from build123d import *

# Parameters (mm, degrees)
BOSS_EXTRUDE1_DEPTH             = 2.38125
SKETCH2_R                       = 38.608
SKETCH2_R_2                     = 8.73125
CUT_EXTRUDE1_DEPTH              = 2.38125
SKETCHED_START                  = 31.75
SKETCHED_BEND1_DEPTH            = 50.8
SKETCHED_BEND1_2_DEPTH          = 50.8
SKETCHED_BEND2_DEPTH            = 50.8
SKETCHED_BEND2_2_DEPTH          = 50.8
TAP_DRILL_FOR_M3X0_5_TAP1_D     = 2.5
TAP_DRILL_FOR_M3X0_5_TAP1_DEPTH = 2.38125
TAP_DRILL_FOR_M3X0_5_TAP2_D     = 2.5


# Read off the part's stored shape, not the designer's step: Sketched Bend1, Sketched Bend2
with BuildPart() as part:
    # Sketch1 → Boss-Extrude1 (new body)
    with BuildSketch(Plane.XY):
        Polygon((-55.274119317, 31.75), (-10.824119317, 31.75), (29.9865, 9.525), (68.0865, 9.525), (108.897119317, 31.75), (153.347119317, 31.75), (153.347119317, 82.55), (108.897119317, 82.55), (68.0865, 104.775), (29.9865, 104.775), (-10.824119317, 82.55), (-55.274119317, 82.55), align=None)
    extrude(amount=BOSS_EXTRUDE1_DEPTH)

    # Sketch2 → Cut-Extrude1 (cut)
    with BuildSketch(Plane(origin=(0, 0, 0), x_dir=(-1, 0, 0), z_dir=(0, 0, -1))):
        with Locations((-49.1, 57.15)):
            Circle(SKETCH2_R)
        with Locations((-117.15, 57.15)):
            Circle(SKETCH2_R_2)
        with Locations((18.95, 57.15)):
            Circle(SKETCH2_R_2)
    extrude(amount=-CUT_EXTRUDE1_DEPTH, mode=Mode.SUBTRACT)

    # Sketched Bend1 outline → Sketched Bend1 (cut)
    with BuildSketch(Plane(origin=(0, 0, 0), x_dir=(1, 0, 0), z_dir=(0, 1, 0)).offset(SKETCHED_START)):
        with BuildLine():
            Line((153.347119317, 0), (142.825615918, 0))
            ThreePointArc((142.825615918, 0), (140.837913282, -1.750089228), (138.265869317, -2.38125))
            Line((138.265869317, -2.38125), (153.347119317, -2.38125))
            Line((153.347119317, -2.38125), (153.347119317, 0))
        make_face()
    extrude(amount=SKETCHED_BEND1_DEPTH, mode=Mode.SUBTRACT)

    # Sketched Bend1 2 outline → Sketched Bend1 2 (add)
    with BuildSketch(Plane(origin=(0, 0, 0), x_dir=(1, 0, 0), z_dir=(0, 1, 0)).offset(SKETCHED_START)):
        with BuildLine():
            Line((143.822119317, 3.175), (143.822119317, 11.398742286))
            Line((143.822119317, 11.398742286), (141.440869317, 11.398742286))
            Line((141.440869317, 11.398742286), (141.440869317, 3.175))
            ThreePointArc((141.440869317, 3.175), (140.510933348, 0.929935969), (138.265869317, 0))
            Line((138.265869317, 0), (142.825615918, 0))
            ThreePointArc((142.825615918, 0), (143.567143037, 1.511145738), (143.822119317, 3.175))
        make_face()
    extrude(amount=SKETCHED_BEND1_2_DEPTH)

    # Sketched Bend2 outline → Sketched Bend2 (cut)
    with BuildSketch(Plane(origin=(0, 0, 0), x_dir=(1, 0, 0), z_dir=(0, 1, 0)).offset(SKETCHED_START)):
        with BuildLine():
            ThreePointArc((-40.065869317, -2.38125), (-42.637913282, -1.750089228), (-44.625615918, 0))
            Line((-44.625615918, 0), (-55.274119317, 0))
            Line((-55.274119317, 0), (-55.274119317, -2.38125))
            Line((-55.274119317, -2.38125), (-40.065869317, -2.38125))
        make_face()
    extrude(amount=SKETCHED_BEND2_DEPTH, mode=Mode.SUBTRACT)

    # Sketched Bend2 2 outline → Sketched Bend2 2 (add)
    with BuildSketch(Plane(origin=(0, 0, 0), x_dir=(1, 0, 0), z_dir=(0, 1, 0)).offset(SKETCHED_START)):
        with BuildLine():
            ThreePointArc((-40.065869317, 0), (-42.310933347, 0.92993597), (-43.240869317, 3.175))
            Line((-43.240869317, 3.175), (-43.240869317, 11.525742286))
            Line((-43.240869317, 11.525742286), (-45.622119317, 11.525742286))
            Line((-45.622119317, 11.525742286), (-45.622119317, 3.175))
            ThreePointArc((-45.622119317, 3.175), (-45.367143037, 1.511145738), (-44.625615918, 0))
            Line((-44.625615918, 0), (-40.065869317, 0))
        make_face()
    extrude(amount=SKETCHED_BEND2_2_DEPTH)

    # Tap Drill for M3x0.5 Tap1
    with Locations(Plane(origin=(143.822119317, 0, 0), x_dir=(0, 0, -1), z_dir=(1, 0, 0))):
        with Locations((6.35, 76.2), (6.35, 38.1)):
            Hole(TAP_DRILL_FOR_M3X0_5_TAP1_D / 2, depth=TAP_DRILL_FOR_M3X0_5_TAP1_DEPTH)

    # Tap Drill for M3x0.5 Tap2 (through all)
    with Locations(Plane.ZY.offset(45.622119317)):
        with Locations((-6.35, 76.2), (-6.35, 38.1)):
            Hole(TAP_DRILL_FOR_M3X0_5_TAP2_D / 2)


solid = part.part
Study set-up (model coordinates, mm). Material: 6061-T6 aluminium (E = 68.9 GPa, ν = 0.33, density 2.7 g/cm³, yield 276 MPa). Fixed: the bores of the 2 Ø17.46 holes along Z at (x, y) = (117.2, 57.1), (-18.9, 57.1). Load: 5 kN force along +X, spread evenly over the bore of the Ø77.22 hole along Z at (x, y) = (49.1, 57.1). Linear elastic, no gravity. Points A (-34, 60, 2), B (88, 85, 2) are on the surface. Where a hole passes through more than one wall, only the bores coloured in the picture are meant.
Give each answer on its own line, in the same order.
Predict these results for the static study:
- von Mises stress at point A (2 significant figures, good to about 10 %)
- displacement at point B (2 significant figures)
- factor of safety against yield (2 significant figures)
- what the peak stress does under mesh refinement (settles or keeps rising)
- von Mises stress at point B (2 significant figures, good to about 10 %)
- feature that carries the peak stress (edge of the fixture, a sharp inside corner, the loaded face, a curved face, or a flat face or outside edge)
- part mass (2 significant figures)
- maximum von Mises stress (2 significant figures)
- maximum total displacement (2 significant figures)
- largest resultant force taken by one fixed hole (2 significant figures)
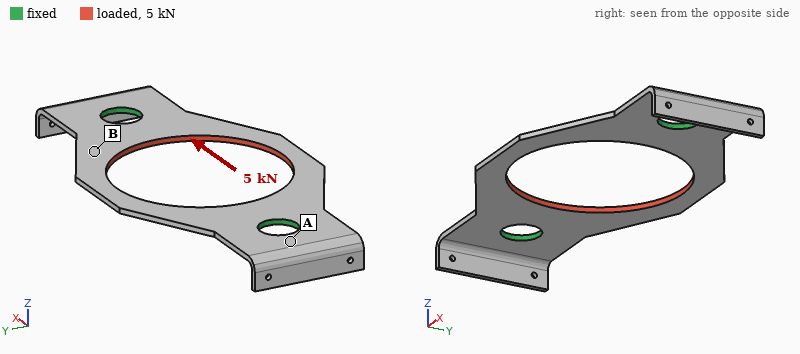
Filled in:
9.2 MPa
24 µm
4.5
settles
28 MPa
a flat face or outside edge
57 g
61 MPa
44 µm
2.5 kN
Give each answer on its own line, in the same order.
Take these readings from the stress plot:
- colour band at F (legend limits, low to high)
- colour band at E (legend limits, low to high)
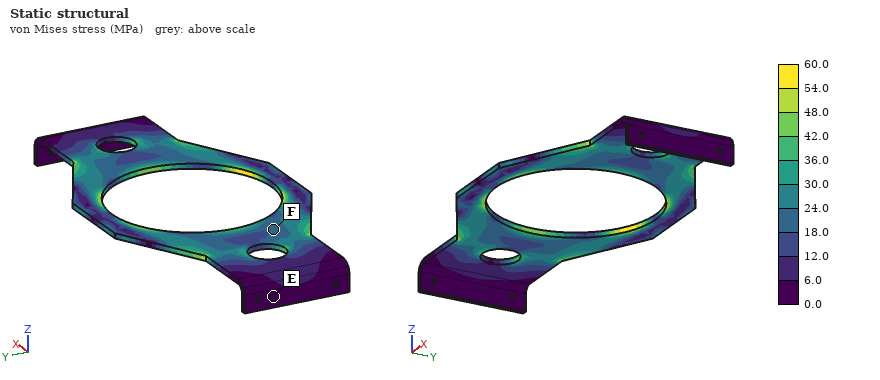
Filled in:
18.0 to 24.0 MPa
0.0 to 6.0 MPa
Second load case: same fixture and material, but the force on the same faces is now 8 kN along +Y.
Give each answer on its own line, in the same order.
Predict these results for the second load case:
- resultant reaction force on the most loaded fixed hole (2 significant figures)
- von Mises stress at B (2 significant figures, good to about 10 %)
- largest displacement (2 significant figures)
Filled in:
4.0 kN
46 MPa
0.11 mm
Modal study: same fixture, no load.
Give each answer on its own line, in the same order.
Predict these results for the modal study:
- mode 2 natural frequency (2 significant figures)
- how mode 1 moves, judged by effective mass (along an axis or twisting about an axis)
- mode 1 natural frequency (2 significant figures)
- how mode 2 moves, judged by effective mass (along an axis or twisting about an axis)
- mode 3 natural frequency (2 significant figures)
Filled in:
700 Hz
twisting about X
670 Hz
along Z
1600 Hz
